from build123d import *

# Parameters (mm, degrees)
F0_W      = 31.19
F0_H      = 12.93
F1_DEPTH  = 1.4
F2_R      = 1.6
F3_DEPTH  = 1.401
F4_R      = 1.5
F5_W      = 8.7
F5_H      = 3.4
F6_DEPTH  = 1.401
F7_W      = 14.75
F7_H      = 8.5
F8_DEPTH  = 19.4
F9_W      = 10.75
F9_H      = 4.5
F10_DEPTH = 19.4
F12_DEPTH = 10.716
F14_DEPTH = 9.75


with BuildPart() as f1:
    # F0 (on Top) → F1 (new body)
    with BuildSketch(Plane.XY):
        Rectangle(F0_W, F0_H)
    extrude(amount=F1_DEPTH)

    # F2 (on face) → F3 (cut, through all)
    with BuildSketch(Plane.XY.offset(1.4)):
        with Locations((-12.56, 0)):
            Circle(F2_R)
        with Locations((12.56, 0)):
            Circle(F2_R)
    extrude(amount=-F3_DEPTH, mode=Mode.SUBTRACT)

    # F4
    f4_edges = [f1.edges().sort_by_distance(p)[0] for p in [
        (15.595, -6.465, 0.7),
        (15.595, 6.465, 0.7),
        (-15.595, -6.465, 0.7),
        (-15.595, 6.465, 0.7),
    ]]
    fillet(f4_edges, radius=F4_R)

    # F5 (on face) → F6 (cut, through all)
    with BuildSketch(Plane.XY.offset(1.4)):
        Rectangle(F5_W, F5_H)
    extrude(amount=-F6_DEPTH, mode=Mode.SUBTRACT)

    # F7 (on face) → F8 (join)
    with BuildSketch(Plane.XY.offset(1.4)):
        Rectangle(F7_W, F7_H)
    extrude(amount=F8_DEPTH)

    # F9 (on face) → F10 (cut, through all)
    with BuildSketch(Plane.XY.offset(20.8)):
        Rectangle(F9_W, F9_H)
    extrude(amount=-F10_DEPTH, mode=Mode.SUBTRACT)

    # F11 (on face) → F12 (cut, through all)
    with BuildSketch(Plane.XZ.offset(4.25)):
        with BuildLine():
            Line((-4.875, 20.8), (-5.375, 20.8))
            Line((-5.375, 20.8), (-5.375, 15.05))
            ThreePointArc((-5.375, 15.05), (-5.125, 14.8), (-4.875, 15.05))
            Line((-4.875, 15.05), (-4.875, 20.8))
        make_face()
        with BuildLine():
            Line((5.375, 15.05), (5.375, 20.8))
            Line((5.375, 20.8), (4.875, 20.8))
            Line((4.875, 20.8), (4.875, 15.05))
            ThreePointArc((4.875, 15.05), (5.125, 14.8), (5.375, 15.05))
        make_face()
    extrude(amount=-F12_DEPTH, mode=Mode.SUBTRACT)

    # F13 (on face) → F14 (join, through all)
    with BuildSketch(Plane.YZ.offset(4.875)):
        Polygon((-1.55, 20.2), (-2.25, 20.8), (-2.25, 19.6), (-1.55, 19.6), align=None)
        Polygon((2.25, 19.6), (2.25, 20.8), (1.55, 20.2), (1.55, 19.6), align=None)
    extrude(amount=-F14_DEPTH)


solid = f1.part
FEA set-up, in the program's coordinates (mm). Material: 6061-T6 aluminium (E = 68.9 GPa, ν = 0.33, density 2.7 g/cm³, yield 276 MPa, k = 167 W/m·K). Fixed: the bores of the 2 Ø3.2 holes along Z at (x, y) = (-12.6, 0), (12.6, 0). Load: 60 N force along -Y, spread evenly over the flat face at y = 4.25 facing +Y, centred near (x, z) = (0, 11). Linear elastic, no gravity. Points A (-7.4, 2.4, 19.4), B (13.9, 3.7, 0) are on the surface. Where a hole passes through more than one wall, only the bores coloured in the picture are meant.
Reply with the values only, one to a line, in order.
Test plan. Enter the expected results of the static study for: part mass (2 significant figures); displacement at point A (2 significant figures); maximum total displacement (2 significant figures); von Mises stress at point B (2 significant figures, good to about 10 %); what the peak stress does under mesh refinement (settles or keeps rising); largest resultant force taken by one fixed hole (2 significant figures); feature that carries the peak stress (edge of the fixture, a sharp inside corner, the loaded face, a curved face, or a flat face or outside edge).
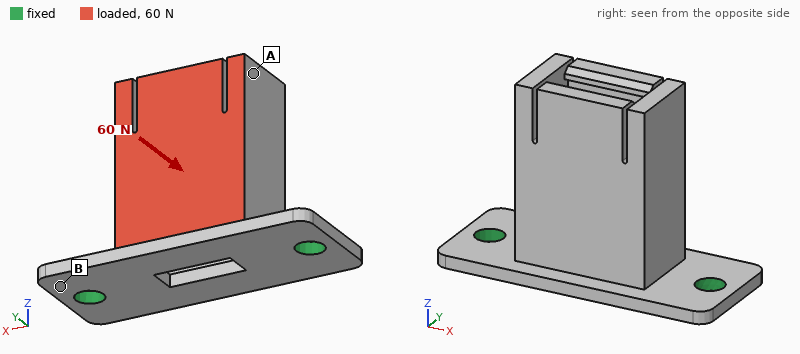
5.3 g
65 µm
75 µm
26 MPa
keeps rising
30 N
edge of the fixture
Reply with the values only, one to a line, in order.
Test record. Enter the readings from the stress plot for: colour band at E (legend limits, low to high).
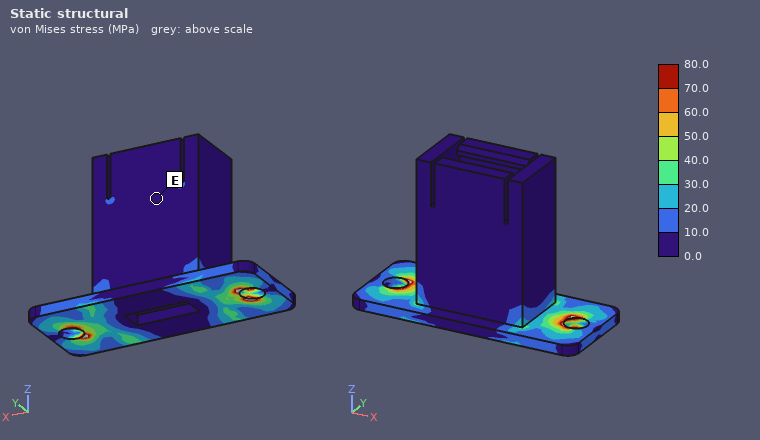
0.0 to 10.0 MPa
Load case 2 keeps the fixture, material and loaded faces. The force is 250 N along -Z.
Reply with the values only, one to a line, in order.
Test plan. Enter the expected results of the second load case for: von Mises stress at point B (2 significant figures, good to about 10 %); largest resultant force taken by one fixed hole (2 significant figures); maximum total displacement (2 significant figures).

58 MPa
140 N
0.13 mm
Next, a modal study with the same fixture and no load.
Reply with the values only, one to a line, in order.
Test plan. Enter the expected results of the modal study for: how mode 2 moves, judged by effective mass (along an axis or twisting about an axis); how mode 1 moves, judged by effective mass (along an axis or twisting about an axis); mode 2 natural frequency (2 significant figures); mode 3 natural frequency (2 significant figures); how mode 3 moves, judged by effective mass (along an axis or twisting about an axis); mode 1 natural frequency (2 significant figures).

along X
along Y
8300 Hz
11 kHz
along Z
2700 Hz
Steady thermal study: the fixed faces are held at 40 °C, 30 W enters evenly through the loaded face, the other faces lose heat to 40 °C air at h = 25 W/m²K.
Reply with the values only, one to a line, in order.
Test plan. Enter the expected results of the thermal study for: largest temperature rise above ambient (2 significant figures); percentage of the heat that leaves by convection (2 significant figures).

67 K
6.6 %
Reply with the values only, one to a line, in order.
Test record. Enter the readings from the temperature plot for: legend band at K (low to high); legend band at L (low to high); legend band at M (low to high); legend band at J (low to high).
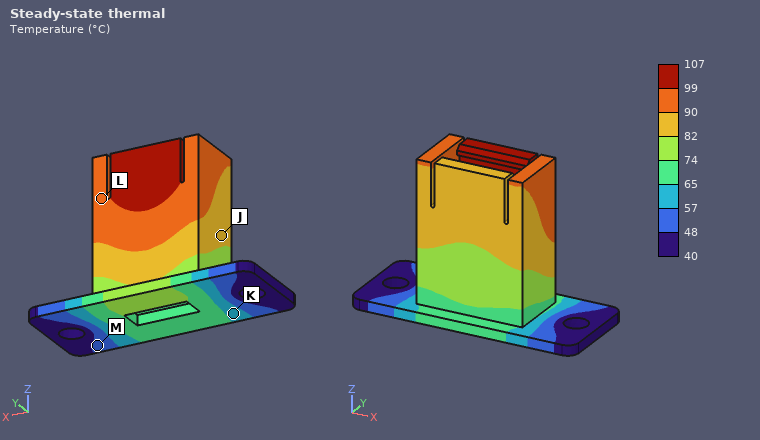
57 to 65 °C
90 to 99 °C
48 to 57 °C
82 to 90 °C
